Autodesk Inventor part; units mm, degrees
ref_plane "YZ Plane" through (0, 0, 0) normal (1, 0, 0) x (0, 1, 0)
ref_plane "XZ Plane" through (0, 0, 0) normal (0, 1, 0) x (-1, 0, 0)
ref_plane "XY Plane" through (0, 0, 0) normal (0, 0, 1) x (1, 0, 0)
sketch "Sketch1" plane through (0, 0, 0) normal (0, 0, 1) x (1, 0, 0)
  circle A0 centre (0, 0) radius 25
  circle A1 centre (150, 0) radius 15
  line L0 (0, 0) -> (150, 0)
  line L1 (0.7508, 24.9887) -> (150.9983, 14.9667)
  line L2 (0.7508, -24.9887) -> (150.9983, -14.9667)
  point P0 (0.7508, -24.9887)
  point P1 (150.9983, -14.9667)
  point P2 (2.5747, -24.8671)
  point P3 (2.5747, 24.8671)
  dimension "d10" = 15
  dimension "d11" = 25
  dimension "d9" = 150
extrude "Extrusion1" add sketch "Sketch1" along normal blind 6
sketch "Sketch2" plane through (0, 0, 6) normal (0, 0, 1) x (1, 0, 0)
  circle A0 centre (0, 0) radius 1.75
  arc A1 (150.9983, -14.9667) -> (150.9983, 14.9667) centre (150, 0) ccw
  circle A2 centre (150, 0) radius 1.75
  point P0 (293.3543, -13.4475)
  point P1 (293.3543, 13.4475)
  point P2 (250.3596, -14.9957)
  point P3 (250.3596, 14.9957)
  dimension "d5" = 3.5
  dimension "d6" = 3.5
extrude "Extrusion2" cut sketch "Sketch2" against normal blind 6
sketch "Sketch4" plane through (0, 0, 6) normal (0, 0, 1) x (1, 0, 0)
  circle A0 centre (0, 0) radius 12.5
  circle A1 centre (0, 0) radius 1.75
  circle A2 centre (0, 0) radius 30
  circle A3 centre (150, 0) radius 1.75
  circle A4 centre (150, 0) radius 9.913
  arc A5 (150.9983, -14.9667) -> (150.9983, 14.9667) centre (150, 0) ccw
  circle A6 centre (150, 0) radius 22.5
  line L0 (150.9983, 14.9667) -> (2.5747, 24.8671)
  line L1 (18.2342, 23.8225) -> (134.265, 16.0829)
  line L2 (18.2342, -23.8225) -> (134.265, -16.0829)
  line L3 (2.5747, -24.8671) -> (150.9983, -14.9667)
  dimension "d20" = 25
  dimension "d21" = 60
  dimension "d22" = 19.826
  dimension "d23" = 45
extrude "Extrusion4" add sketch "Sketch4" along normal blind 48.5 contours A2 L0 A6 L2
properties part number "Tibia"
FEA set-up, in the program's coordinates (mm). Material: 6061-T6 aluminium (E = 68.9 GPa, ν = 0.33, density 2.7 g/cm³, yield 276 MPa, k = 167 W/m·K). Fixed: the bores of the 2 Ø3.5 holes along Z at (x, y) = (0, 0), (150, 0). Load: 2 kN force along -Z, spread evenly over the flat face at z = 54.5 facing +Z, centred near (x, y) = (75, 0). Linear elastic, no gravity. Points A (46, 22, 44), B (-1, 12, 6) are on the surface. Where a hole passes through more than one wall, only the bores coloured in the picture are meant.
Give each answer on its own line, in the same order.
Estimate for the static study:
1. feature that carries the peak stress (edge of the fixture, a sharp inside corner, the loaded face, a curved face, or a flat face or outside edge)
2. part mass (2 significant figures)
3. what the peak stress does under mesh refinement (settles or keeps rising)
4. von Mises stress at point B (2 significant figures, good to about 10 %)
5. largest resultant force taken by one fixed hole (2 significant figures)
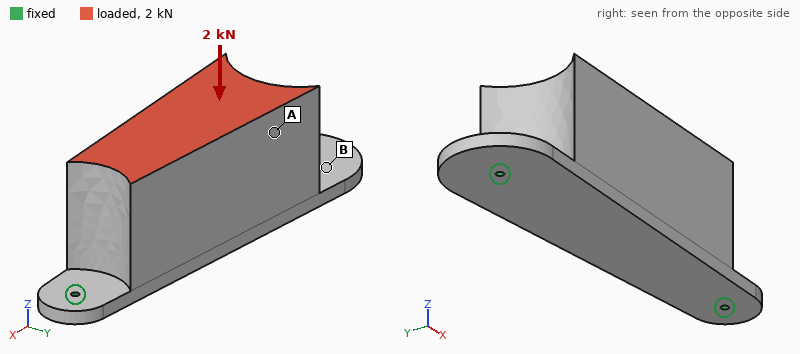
edge of the fixture
650 g
keeps rising
15 MPa
1.2 kN
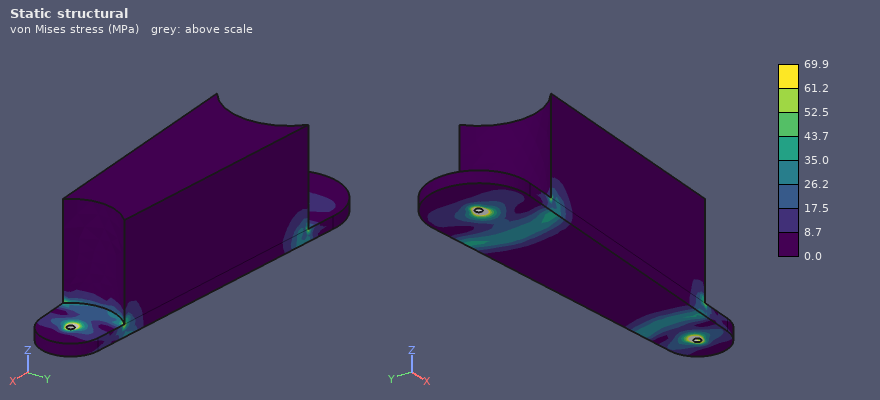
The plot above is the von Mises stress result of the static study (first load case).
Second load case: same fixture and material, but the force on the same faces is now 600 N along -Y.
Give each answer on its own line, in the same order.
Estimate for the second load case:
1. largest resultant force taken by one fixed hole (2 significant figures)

300 N
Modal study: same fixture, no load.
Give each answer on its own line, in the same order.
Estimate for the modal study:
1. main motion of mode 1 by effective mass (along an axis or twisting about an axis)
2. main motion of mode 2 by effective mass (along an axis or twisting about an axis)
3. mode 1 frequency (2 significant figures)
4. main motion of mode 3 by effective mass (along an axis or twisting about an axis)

along Y
along Z
490 Hz
along X
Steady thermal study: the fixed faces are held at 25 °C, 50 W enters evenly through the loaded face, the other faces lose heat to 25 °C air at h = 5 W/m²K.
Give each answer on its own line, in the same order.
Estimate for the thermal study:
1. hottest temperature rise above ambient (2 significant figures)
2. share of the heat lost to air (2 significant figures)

27 K
5.8 %
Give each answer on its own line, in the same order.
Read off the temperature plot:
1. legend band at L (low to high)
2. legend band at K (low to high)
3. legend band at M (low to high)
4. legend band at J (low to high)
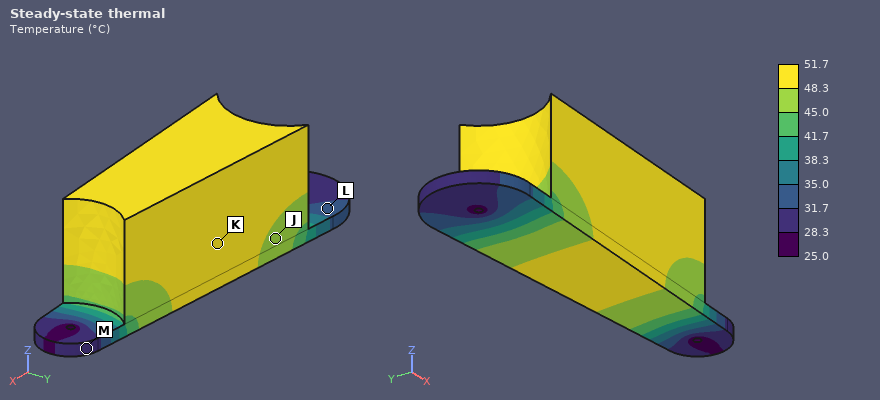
31.7 to 35.0 °C
48.3 to 51.7 °C
28.3 to 31.7 °C
45.0 to 48.3 °C
